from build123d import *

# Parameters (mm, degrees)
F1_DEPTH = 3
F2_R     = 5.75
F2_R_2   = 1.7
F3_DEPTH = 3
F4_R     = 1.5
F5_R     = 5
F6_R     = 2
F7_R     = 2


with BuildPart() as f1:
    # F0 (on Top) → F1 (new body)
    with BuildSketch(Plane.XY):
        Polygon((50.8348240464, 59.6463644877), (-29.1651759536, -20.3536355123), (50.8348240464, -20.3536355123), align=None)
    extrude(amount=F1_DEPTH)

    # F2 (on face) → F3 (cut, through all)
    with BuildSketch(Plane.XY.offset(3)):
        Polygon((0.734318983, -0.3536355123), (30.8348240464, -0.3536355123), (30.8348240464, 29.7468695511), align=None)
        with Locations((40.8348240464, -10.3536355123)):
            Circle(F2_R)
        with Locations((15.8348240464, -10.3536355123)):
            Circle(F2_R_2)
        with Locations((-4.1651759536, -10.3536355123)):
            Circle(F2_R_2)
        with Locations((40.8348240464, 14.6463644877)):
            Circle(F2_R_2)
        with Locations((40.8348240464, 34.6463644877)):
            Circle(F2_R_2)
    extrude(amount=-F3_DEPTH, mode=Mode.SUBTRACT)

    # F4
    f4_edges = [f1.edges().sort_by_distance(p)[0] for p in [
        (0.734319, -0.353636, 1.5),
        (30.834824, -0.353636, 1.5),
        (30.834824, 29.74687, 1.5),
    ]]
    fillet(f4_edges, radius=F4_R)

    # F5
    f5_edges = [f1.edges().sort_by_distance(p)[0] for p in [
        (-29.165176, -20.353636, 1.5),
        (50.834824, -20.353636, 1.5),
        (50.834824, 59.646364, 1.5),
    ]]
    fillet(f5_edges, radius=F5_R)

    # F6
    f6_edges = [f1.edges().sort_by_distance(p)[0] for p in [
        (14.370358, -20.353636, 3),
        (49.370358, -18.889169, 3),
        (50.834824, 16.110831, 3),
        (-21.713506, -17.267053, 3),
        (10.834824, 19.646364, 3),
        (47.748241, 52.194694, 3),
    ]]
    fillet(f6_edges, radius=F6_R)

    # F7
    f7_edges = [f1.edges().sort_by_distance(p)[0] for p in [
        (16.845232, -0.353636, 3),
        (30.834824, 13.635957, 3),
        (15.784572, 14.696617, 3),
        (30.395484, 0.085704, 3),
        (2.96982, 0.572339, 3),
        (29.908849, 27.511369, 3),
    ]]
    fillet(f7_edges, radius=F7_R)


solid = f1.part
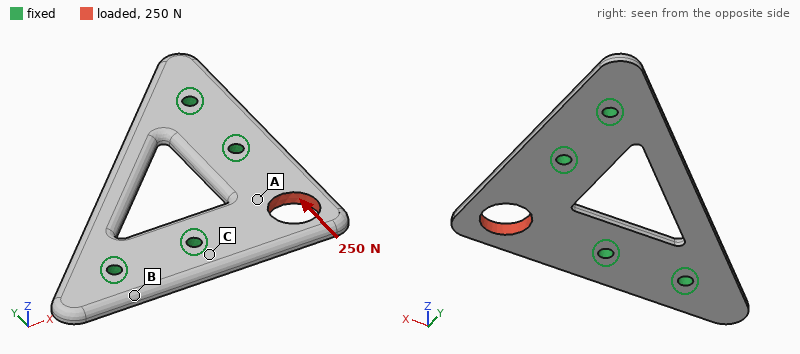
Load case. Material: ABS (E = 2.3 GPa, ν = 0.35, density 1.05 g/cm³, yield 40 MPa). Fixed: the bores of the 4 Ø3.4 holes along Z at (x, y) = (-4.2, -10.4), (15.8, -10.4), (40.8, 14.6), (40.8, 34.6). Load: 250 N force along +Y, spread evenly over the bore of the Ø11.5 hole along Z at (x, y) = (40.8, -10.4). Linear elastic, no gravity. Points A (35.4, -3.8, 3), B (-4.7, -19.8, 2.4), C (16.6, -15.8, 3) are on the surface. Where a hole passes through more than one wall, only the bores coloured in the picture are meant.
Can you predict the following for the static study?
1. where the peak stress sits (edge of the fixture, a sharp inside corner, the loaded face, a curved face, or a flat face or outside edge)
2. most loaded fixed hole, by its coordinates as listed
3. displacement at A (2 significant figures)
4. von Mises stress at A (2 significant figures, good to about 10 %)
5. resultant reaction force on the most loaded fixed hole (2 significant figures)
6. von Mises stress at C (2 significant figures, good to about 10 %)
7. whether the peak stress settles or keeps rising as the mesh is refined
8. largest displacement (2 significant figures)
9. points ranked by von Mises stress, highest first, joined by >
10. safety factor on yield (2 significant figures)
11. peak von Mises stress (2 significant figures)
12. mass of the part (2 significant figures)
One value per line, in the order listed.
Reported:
the loaded face
(40.8, 14.6)
0.035 mm
5.4 MPa
180 N
1.5 MPa
settles
0.10 mm
A > C > B
3.1
13 MPa
7.7 g
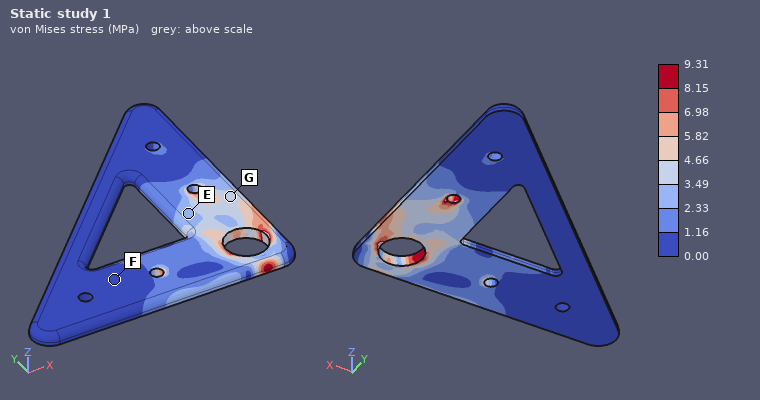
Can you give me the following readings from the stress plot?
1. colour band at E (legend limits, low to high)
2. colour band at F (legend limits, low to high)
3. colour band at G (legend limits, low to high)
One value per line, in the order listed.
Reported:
2.33 to 3.49 MPa
0.00 to 1.16 MPa
3.49 to 4.66 MPa
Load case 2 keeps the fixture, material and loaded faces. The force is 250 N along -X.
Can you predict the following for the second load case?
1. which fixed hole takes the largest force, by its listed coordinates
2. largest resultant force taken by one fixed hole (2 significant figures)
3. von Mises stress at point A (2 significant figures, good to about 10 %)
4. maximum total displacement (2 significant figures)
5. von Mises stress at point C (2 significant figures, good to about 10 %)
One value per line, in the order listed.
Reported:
(15.8, -10.4)
180 N
5.0 MPa
0.10 mm
2.5 MPa
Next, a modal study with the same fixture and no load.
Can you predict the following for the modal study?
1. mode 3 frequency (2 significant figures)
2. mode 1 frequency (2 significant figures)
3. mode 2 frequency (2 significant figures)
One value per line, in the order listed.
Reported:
2900 Hz
1200 Hz
1400 Hz
